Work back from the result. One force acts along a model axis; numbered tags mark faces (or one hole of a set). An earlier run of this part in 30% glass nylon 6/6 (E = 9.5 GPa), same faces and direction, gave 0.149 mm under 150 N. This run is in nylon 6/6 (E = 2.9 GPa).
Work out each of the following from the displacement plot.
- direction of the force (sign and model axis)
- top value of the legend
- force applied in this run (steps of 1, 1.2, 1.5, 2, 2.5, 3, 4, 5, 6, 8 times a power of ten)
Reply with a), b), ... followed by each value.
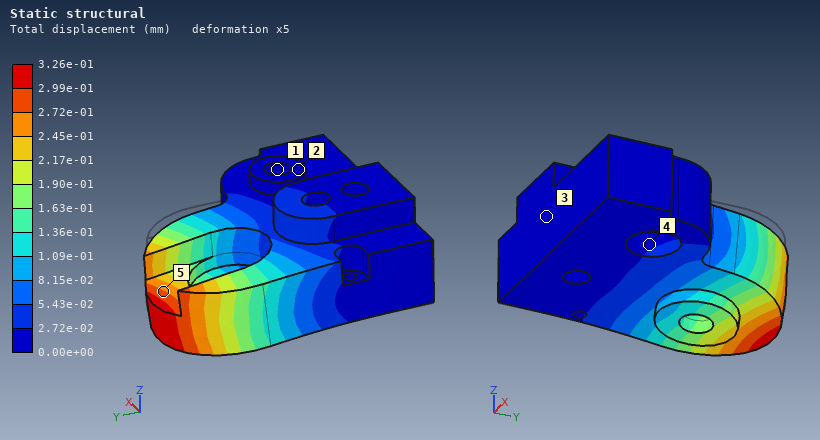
a) -Z
b) 3.26e-01 mm
c) 100 N
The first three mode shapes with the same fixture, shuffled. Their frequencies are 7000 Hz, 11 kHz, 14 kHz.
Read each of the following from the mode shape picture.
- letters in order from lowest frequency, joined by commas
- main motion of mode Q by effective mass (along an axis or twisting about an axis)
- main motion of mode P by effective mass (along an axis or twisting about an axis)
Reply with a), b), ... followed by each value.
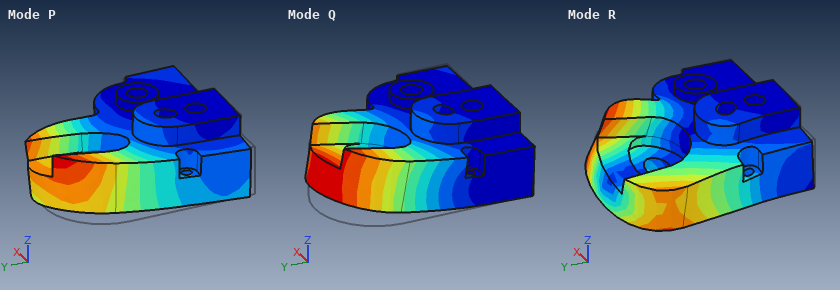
a) Q, P, R
b) along Z
c) along X
